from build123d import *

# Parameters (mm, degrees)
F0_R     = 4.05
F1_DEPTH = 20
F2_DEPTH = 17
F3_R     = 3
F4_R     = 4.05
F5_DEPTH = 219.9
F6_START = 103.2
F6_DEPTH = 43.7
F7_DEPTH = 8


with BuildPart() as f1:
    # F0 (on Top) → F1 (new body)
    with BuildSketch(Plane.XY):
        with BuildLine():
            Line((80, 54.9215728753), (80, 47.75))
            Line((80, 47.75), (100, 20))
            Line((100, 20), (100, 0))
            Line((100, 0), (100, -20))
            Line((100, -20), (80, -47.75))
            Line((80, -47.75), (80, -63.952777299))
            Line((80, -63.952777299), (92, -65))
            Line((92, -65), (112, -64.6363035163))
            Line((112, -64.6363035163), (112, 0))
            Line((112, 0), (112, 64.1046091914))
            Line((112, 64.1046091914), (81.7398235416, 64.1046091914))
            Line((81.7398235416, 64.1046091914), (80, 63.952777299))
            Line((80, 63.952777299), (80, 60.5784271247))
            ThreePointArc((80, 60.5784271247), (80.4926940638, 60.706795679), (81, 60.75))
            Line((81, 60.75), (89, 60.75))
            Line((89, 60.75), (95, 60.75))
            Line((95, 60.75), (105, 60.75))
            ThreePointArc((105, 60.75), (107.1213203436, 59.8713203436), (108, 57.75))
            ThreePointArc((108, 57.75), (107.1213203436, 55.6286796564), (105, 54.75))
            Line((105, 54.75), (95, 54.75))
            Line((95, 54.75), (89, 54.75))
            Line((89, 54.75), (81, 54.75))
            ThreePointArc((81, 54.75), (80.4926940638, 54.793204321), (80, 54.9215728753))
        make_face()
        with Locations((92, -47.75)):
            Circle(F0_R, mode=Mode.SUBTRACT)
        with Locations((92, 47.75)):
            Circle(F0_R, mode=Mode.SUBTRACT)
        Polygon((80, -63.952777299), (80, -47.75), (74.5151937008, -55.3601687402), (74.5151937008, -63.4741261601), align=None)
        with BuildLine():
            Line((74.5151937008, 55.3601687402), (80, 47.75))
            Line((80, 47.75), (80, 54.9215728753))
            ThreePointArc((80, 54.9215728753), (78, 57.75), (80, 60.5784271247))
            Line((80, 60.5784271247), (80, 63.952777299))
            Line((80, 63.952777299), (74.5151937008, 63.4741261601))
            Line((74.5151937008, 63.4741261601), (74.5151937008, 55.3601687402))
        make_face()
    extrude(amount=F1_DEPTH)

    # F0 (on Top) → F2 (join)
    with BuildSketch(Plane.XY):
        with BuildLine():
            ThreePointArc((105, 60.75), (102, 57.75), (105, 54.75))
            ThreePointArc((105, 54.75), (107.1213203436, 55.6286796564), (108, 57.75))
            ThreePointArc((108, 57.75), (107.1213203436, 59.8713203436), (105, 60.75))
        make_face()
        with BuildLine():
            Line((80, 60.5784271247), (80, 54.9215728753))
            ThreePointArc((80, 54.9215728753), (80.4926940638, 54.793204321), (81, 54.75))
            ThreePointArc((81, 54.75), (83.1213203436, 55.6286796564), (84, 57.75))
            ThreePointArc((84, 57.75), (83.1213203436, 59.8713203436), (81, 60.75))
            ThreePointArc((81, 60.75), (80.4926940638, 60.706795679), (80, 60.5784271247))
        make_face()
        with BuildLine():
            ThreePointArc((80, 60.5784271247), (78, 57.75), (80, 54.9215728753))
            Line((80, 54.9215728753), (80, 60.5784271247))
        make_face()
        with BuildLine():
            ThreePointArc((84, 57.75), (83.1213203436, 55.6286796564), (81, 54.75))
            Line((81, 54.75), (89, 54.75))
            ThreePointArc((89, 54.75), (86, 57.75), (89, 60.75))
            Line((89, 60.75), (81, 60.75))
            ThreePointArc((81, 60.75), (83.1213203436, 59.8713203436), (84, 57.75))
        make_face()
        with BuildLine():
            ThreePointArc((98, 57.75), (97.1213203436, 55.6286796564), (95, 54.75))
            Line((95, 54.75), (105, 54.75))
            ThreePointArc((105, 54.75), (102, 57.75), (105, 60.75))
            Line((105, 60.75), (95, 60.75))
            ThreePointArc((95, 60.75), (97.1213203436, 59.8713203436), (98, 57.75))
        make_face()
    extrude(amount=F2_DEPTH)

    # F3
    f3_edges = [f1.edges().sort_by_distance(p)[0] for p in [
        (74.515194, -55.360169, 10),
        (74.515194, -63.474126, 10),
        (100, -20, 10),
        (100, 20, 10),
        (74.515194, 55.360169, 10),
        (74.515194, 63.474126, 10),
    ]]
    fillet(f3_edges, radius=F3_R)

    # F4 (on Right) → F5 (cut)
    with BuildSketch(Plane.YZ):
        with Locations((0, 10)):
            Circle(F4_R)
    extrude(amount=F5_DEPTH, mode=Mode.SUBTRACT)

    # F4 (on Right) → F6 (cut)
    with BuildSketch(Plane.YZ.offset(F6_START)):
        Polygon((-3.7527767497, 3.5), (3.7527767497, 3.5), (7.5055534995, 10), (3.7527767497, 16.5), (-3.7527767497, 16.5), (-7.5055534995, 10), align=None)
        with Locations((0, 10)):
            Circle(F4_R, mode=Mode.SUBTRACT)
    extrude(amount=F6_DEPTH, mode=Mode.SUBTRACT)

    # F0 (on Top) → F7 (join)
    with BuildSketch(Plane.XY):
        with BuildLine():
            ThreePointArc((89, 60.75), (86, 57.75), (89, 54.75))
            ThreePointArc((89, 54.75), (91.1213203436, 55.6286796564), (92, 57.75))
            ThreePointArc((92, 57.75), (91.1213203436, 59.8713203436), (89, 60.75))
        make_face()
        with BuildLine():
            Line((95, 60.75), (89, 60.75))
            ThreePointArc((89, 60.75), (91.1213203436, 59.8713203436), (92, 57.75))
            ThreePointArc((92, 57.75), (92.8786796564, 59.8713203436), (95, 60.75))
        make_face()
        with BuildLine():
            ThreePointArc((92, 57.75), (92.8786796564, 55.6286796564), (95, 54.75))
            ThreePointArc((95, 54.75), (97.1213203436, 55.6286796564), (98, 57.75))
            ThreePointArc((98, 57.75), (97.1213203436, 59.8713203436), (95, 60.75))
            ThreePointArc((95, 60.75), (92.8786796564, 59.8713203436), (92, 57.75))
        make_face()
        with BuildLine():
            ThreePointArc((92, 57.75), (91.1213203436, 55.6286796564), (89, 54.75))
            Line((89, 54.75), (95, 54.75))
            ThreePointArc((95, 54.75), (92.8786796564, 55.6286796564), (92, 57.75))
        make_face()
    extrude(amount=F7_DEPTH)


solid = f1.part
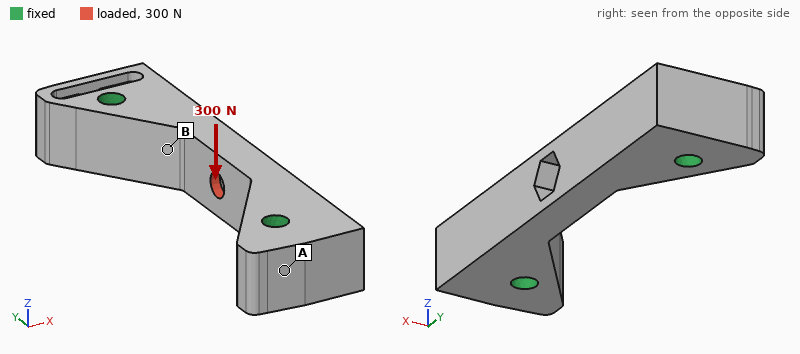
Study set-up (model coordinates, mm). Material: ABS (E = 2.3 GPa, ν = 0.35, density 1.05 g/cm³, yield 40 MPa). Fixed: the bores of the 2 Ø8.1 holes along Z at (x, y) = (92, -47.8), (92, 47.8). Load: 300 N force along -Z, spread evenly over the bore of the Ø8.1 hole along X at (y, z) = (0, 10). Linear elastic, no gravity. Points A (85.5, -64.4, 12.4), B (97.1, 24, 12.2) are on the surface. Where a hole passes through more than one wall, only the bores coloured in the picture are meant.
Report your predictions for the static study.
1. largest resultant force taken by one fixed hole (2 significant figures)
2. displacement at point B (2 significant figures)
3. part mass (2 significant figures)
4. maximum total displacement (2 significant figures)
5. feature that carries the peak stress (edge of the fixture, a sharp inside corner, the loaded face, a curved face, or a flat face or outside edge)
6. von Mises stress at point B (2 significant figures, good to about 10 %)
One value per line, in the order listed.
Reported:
150 N
0.040 mm
56 g
0.12 mm
a sharp inside corner
2.4 MPa
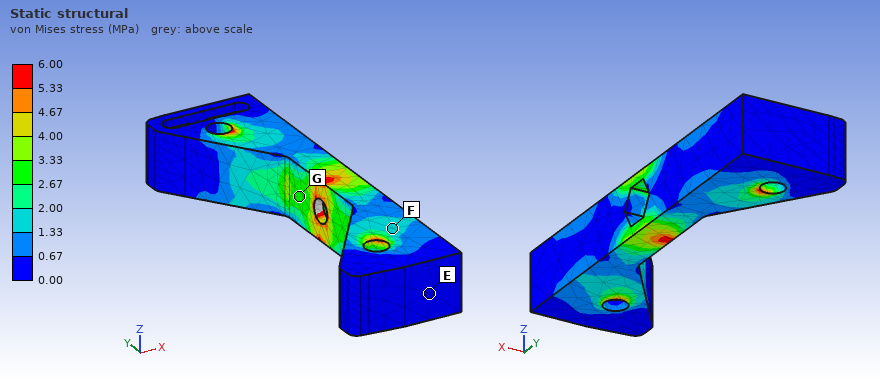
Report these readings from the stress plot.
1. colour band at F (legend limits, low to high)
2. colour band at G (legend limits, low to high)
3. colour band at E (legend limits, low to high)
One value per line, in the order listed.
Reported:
1.33 to 2.00 MPa
2.67 to 3.33 MPa
0.00 to 0.67 MPa
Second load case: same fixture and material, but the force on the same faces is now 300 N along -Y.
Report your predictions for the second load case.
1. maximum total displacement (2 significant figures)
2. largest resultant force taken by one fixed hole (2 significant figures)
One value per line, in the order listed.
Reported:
32 µm
150 N
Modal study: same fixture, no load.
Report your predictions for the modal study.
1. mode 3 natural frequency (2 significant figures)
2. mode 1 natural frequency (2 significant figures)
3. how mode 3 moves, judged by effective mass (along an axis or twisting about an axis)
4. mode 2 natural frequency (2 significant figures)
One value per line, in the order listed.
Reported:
3800 Hz
2900 Hz
along Y
3000 Hz
